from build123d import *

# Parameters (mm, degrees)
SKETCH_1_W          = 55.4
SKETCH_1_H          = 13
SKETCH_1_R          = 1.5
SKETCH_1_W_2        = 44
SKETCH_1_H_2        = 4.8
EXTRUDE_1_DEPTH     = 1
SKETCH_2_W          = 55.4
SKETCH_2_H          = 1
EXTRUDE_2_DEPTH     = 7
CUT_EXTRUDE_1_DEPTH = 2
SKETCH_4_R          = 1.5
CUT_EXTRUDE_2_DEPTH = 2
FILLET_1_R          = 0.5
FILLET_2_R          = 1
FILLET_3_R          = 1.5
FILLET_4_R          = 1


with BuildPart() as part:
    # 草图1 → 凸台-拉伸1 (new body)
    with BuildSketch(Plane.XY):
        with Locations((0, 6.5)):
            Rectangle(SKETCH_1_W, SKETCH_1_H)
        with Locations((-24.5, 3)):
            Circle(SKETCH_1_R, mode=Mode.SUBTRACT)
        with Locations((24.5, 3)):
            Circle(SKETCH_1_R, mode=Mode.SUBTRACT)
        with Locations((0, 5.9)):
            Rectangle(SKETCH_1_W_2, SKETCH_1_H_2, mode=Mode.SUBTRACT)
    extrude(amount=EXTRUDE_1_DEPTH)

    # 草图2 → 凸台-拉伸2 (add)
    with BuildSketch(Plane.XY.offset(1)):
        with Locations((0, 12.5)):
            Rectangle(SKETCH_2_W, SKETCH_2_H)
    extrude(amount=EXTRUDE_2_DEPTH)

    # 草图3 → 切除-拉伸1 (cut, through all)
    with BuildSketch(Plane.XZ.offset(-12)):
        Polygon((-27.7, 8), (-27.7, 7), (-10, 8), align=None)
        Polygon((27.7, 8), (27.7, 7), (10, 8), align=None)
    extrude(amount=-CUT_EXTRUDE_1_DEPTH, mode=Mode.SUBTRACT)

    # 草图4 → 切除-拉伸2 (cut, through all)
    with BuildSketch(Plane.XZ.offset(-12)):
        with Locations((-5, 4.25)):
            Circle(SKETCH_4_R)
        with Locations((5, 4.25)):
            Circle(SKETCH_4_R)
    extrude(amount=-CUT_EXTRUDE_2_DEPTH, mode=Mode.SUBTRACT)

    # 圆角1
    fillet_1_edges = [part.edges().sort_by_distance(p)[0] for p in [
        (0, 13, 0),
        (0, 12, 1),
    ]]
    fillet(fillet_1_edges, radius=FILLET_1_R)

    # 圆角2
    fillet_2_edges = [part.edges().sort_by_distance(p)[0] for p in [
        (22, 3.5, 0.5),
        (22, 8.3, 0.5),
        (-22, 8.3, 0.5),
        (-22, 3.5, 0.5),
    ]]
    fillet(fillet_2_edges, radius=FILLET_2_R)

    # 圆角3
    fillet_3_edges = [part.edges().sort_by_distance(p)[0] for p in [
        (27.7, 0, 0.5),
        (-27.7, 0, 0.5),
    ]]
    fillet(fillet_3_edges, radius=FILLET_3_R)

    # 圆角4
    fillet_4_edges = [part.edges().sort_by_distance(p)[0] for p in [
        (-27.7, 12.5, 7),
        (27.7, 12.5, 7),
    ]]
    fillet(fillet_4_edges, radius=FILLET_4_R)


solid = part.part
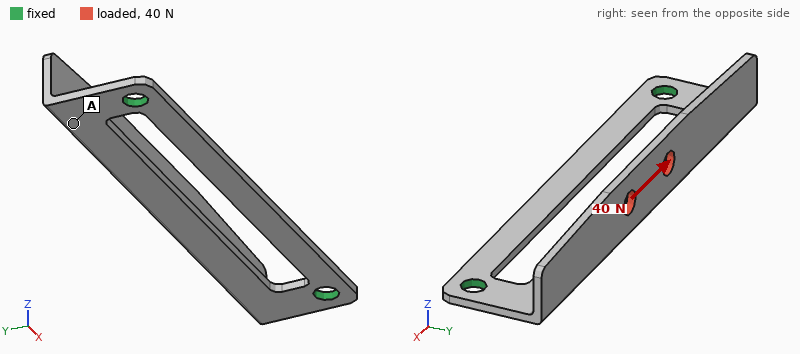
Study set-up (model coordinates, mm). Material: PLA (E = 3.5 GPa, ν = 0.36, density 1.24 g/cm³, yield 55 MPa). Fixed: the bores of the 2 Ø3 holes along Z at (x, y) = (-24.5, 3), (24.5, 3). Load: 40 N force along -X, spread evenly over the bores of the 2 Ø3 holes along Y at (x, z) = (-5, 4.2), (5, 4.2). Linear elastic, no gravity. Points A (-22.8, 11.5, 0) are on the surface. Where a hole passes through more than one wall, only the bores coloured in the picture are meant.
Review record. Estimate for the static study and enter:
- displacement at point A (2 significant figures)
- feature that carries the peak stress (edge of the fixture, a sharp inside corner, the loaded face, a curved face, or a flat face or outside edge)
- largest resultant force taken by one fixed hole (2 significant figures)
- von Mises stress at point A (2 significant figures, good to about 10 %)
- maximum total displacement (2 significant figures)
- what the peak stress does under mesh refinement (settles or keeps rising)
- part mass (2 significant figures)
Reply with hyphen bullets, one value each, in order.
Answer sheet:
- 0.17 mm
- edge of the fixture
- 20 N
- 4.1 MPa
- 0.32 mm
- keeps rising
- 1.1 g
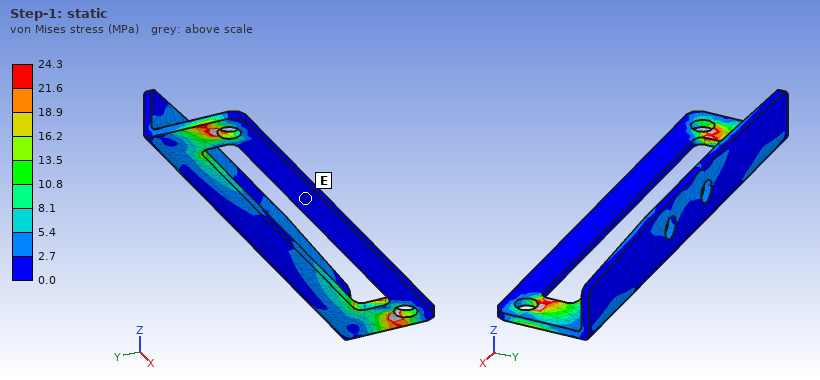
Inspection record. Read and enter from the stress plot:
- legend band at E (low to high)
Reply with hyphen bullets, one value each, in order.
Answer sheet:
- 0.0 to 2.7 MPa
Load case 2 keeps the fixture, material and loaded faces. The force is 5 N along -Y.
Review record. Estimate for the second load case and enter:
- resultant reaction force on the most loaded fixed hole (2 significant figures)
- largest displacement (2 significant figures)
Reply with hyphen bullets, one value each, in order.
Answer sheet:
- 4.3 N
- 0.63 mm
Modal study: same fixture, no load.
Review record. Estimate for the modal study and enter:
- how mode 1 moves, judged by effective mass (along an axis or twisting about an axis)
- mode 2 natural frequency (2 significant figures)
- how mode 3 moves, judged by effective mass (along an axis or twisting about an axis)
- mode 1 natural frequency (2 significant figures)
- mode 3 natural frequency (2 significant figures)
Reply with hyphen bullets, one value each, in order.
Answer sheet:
- along Z
- 810 Hz
- twisting about Y
- 710 Hz
- 1400 Hz
